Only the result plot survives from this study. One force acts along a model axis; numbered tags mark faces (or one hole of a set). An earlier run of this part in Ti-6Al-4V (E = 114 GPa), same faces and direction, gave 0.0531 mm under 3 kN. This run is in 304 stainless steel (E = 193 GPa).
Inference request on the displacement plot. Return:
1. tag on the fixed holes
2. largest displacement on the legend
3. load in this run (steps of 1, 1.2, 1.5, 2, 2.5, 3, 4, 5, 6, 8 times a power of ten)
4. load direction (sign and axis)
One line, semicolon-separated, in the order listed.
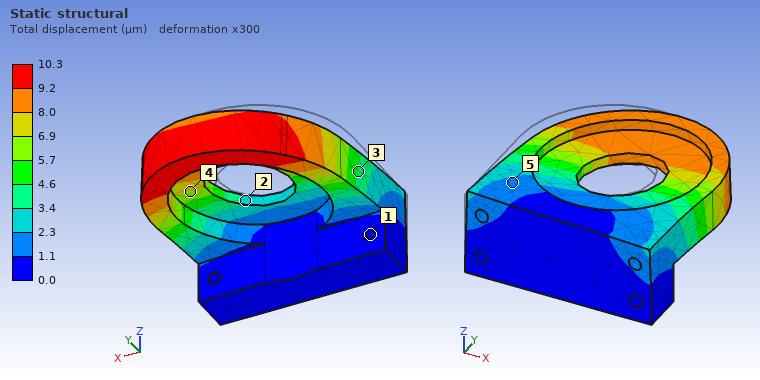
1; 10.3 µm; 1 kN; +X
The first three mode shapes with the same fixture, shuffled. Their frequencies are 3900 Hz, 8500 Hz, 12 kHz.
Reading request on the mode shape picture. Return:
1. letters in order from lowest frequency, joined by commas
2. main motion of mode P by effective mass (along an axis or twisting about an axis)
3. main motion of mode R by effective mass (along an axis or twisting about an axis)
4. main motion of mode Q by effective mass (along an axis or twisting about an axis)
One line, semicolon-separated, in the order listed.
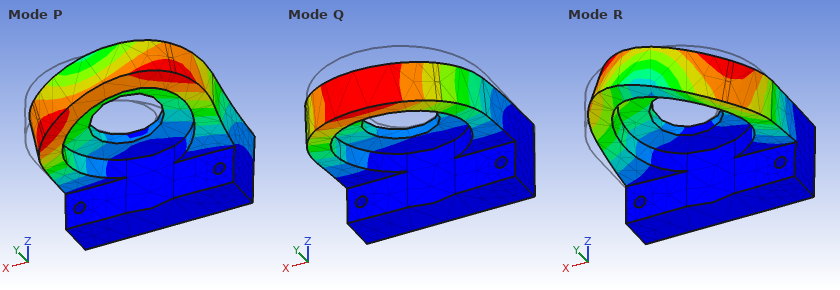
Q, P, R; along X; along X; along Z
